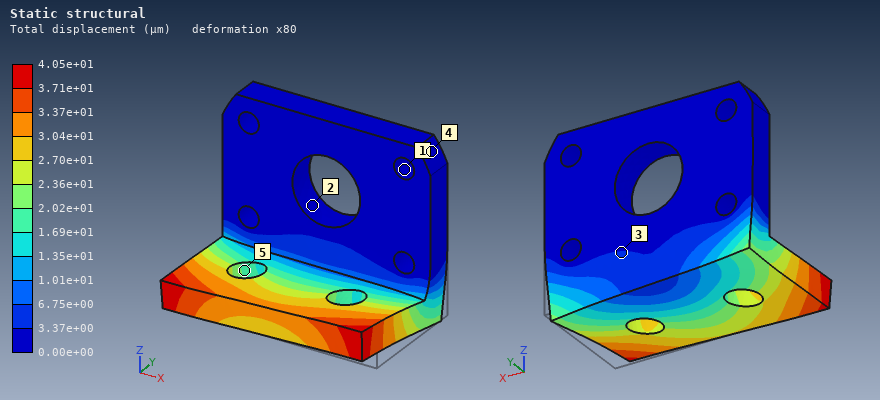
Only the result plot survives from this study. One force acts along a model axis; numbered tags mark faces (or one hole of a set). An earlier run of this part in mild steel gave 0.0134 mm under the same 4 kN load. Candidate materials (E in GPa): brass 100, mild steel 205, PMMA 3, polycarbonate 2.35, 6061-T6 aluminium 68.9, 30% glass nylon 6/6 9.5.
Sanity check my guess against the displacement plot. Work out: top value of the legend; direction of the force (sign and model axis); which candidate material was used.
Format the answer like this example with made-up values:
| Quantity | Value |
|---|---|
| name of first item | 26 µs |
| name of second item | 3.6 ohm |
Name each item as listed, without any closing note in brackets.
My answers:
| Quantity | Value |
|---|---|
| top value of the legend | 4.05e+01 µm |
| direction of the force | -X |
| which candidate material was used | 6061-T6 aluminium |
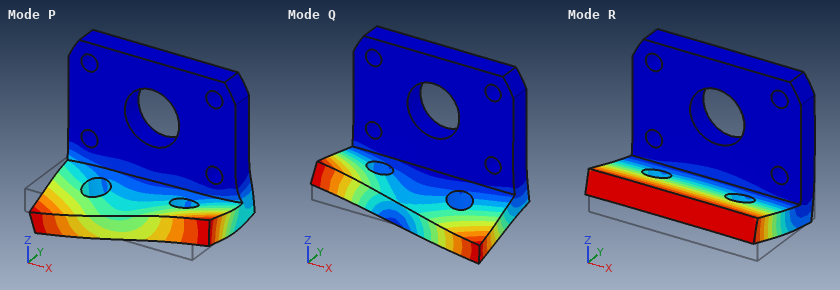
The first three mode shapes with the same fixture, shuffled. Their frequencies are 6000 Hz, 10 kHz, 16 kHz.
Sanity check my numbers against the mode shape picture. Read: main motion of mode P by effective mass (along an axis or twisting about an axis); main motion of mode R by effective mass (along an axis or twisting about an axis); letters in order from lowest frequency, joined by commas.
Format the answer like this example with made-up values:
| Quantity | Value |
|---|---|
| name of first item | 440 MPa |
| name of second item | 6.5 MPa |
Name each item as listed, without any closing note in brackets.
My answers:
| Quantity | Value |
|---|---|
| main motion of mode P by effective mass | along X |
| main motion of mode R by effective mass | along Z |
| letters in order from lowest frequency, joined by commas | R, Q, P |
